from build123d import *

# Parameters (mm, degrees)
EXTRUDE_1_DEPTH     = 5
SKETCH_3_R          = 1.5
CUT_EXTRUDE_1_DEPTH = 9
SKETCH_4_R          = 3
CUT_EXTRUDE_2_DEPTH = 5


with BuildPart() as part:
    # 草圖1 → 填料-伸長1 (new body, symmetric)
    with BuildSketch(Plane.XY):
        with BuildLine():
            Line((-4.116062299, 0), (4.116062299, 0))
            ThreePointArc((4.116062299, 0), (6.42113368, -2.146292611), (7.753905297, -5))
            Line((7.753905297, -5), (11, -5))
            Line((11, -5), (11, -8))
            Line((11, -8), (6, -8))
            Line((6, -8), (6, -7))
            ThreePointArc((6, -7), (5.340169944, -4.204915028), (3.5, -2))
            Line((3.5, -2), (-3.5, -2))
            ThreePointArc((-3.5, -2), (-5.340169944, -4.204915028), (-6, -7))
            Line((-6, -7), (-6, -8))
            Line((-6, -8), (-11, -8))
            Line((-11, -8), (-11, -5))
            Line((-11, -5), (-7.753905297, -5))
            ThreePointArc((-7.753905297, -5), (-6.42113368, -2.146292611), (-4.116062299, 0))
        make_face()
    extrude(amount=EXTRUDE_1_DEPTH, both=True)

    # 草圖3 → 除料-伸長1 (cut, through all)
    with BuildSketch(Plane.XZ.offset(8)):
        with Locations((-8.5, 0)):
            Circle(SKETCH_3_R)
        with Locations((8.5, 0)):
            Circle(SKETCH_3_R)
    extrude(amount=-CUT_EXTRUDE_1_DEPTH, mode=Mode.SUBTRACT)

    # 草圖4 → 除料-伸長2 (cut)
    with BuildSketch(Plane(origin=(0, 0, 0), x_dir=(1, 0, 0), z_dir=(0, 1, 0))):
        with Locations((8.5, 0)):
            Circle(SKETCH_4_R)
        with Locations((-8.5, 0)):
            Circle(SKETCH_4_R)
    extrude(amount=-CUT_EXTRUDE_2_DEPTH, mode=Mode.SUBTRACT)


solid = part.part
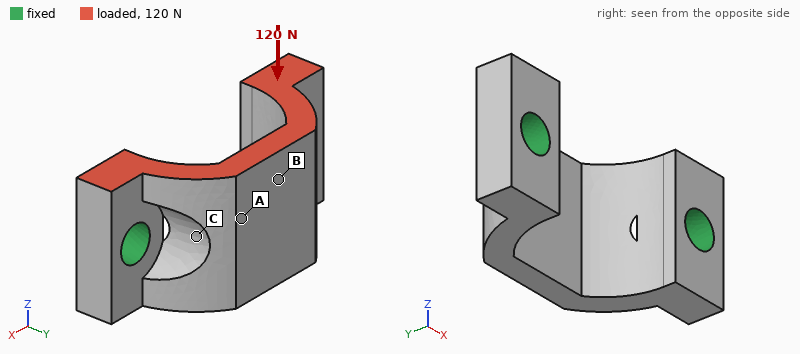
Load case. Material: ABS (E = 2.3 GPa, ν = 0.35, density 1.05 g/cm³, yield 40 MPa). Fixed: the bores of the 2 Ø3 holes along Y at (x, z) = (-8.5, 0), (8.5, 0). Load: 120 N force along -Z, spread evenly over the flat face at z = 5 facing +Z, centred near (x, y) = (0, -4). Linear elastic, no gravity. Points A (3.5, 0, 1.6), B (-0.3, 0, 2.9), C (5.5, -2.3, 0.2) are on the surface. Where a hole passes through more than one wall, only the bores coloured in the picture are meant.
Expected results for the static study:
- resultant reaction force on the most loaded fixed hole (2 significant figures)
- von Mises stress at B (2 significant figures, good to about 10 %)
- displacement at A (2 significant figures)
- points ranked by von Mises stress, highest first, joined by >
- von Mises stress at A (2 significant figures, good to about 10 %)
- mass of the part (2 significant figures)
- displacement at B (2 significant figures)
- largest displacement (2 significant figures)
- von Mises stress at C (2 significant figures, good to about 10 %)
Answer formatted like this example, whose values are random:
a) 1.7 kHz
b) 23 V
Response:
a) 60 N
b) 1.8 MPa
c) 58 µm
d) C > A > B
e) 3.3 MPa
f) 0.60 g
g) 63 µm
h) 70 µm
i) 6.5 MPa
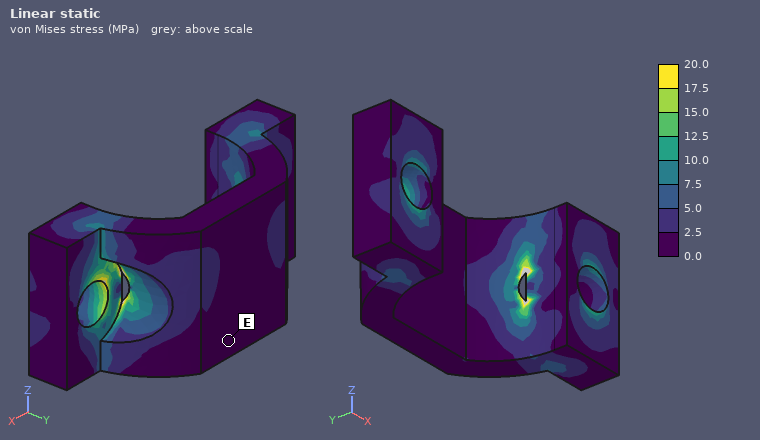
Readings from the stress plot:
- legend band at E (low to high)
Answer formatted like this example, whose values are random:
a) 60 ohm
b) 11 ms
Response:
a) 0.0 to 2.5 MPa
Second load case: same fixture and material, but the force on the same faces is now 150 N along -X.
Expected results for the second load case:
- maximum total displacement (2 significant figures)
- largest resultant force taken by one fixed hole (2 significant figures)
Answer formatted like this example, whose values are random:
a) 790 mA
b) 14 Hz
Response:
a) 0.12 mm
b) 80 N
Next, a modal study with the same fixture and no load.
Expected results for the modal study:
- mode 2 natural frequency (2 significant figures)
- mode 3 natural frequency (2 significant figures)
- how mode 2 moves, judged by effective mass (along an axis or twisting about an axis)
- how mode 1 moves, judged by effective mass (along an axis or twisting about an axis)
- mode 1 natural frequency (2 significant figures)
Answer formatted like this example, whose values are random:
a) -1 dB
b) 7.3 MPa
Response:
a) 10 kHz
b) 14 kHz
c) along X
d) along Z
e) 9300 Hz
